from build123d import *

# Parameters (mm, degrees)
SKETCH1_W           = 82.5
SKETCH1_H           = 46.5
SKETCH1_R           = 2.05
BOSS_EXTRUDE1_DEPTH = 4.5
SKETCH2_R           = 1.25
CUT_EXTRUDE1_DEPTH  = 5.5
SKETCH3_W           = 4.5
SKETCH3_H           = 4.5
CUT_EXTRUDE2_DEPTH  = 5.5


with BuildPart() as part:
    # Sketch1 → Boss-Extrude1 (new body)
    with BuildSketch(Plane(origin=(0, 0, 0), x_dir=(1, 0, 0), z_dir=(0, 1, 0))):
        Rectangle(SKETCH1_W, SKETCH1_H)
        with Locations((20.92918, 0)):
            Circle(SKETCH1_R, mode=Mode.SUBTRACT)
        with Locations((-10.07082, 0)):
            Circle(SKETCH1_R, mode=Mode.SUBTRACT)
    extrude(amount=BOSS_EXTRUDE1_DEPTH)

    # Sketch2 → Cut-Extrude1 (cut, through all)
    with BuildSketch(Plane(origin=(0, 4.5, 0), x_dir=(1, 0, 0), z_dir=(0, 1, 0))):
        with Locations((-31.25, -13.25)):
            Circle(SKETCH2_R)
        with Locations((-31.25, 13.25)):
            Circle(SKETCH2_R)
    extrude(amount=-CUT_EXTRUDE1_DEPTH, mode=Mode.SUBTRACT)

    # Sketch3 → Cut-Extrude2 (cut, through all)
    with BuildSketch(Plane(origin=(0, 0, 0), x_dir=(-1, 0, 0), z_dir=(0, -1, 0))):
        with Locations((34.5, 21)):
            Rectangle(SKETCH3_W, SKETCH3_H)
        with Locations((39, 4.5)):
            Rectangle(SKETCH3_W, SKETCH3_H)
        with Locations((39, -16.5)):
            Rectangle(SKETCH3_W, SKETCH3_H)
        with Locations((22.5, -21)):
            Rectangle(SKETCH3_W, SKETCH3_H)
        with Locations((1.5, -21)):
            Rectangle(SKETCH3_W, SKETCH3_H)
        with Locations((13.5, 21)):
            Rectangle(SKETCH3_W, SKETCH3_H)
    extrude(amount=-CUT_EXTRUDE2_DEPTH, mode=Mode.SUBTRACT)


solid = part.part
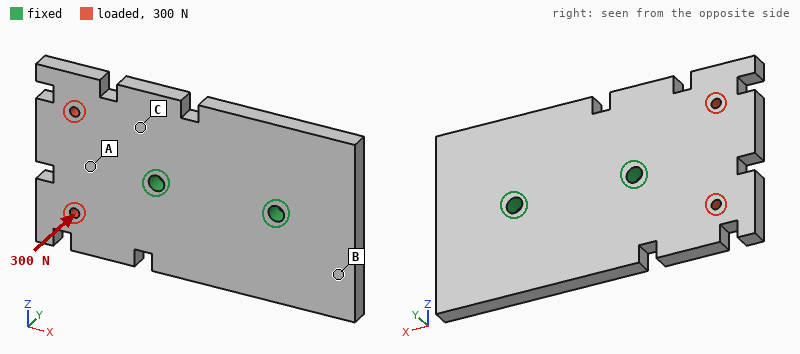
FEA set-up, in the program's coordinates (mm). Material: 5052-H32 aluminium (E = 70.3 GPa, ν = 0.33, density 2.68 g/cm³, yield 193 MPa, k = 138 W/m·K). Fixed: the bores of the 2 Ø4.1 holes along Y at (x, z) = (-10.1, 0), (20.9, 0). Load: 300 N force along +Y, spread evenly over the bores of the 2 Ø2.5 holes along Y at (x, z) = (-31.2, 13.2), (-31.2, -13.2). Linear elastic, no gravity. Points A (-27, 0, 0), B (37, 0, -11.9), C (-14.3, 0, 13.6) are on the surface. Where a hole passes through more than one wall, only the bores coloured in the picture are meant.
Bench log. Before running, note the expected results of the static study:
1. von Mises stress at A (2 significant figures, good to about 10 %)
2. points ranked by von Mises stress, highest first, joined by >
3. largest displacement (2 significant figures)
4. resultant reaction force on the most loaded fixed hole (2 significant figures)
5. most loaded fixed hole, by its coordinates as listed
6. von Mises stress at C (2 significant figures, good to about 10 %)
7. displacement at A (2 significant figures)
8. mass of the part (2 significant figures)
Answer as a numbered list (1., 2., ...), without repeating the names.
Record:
1. 13 MPa
2. C > A > B
3. 97 µm
4. 380 N
5. (-10.1, 0)
6. 23 MPa
7. 41 µm
8. 44 g
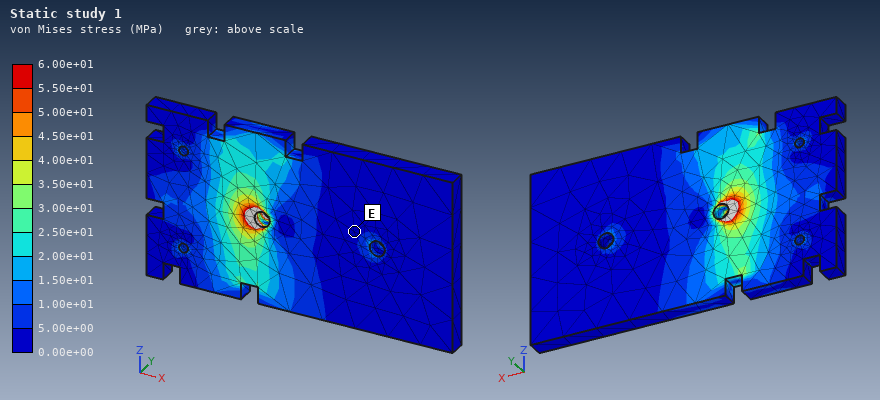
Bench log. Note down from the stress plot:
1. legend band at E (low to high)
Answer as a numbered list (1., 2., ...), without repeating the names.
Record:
1. 0.00e+00 to 5.00e+00 MPa
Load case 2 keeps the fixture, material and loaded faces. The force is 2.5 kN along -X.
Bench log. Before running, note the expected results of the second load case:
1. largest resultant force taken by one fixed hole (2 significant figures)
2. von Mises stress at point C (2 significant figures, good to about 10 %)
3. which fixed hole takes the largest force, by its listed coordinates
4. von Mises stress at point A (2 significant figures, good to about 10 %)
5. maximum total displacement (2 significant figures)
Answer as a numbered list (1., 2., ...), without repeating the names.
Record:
1. 1.8 kN
2. 12 MPa
3. (-10.1, 0)
4. 7.8 MPa
5. 9.7 µm
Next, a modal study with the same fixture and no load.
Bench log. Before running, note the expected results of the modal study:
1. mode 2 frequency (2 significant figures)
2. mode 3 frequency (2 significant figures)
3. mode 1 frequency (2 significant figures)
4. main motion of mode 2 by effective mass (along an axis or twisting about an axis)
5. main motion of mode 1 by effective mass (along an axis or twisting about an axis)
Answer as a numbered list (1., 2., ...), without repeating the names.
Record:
1. 4100 Hz
2. 5200 Hz
3. 3400 Hz
4. twisting about X
5. along Y
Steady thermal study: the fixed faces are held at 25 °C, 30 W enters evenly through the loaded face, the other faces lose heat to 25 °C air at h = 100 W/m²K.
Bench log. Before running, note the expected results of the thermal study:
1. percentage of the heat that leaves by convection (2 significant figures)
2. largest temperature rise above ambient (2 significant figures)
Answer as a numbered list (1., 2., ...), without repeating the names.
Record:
1. 26 %
2. 32 K
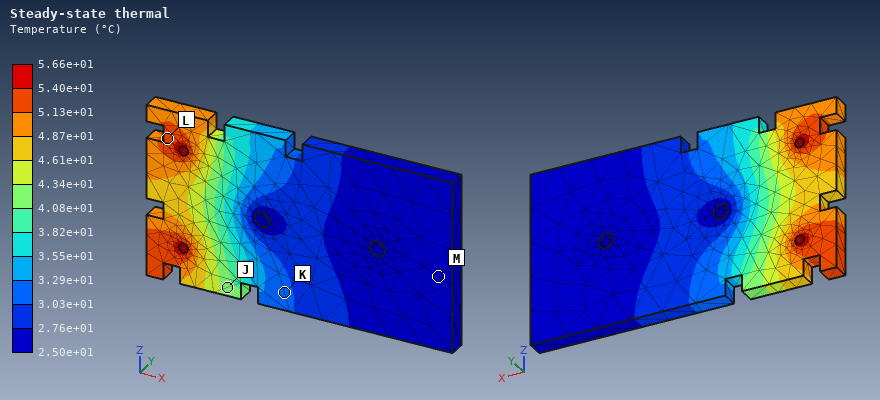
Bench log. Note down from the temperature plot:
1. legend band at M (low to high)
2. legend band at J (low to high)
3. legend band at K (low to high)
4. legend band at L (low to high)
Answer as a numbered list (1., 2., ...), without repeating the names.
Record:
1. 2.50e+01 to 2.76e+01 °C
2. 4.08e+01 to 4.34e+01 °C
3. 3.03e+01 to 3.29e+01 °C
4. 5.13e+01 to 5.40e+01 °C
